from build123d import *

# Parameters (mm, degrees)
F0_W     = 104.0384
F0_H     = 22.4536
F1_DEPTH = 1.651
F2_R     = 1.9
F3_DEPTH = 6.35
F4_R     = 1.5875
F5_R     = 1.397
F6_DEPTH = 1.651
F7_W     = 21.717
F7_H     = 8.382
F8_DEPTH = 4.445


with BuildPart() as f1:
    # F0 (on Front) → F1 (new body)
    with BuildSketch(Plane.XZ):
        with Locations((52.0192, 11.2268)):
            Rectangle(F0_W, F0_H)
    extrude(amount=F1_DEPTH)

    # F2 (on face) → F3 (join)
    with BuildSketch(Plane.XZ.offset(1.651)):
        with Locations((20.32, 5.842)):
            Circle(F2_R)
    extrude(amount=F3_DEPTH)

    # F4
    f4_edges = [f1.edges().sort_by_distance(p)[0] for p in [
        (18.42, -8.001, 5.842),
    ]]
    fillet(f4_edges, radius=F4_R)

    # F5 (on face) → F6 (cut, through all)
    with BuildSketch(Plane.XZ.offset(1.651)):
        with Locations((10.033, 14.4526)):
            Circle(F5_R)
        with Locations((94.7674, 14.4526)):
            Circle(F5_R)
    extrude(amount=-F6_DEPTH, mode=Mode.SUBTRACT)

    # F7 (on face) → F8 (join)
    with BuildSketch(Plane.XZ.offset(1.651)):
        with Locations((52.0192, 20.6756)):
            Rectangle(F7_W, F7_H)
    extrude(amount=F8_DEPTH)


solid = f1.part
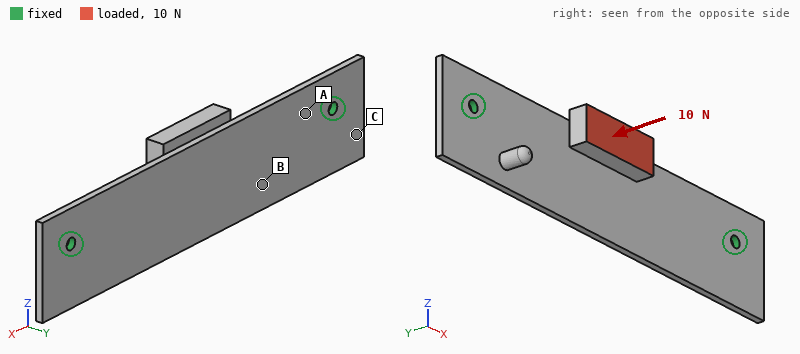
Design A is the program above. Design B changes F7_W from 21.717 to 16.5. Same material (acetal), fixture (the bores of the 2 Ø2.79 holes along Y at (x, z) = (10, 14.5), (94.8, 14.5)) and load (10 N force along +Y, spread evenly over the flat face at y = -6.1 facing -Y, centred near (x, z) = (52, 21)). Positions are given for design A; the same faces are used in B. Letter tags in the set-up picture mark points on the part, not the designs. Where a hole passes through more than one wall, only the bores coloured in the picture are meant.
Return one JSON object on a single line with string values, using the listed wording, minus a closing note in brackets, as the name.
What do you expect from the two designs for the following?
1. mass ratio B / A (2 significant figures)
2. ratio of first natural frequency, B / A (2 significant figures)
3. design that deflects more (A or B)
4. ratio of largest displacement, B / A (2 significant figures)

{"mass ratio B / A": "0.96", "ratio of first natural frequency, B / A": "0.97", "design that deflects more": "B", "ratio of largest displacement, B / A": "1.2"}
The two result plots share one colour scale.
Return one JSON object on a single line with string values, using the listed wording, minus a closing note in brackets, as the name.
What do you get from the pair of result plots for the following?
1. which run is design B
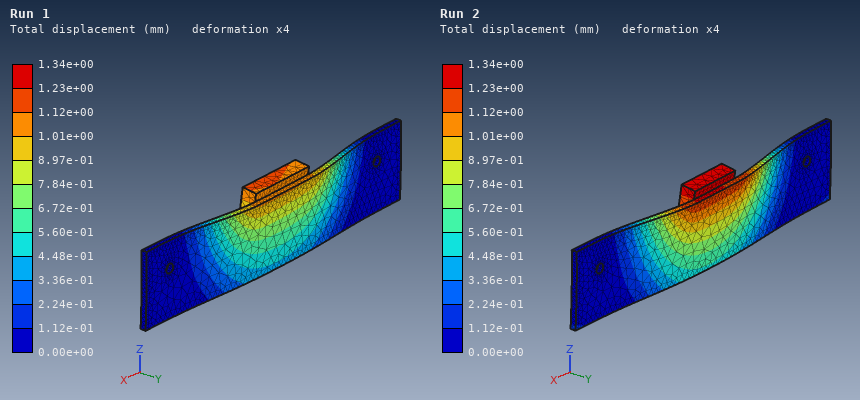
{"which run is design B": "Run 2"}
